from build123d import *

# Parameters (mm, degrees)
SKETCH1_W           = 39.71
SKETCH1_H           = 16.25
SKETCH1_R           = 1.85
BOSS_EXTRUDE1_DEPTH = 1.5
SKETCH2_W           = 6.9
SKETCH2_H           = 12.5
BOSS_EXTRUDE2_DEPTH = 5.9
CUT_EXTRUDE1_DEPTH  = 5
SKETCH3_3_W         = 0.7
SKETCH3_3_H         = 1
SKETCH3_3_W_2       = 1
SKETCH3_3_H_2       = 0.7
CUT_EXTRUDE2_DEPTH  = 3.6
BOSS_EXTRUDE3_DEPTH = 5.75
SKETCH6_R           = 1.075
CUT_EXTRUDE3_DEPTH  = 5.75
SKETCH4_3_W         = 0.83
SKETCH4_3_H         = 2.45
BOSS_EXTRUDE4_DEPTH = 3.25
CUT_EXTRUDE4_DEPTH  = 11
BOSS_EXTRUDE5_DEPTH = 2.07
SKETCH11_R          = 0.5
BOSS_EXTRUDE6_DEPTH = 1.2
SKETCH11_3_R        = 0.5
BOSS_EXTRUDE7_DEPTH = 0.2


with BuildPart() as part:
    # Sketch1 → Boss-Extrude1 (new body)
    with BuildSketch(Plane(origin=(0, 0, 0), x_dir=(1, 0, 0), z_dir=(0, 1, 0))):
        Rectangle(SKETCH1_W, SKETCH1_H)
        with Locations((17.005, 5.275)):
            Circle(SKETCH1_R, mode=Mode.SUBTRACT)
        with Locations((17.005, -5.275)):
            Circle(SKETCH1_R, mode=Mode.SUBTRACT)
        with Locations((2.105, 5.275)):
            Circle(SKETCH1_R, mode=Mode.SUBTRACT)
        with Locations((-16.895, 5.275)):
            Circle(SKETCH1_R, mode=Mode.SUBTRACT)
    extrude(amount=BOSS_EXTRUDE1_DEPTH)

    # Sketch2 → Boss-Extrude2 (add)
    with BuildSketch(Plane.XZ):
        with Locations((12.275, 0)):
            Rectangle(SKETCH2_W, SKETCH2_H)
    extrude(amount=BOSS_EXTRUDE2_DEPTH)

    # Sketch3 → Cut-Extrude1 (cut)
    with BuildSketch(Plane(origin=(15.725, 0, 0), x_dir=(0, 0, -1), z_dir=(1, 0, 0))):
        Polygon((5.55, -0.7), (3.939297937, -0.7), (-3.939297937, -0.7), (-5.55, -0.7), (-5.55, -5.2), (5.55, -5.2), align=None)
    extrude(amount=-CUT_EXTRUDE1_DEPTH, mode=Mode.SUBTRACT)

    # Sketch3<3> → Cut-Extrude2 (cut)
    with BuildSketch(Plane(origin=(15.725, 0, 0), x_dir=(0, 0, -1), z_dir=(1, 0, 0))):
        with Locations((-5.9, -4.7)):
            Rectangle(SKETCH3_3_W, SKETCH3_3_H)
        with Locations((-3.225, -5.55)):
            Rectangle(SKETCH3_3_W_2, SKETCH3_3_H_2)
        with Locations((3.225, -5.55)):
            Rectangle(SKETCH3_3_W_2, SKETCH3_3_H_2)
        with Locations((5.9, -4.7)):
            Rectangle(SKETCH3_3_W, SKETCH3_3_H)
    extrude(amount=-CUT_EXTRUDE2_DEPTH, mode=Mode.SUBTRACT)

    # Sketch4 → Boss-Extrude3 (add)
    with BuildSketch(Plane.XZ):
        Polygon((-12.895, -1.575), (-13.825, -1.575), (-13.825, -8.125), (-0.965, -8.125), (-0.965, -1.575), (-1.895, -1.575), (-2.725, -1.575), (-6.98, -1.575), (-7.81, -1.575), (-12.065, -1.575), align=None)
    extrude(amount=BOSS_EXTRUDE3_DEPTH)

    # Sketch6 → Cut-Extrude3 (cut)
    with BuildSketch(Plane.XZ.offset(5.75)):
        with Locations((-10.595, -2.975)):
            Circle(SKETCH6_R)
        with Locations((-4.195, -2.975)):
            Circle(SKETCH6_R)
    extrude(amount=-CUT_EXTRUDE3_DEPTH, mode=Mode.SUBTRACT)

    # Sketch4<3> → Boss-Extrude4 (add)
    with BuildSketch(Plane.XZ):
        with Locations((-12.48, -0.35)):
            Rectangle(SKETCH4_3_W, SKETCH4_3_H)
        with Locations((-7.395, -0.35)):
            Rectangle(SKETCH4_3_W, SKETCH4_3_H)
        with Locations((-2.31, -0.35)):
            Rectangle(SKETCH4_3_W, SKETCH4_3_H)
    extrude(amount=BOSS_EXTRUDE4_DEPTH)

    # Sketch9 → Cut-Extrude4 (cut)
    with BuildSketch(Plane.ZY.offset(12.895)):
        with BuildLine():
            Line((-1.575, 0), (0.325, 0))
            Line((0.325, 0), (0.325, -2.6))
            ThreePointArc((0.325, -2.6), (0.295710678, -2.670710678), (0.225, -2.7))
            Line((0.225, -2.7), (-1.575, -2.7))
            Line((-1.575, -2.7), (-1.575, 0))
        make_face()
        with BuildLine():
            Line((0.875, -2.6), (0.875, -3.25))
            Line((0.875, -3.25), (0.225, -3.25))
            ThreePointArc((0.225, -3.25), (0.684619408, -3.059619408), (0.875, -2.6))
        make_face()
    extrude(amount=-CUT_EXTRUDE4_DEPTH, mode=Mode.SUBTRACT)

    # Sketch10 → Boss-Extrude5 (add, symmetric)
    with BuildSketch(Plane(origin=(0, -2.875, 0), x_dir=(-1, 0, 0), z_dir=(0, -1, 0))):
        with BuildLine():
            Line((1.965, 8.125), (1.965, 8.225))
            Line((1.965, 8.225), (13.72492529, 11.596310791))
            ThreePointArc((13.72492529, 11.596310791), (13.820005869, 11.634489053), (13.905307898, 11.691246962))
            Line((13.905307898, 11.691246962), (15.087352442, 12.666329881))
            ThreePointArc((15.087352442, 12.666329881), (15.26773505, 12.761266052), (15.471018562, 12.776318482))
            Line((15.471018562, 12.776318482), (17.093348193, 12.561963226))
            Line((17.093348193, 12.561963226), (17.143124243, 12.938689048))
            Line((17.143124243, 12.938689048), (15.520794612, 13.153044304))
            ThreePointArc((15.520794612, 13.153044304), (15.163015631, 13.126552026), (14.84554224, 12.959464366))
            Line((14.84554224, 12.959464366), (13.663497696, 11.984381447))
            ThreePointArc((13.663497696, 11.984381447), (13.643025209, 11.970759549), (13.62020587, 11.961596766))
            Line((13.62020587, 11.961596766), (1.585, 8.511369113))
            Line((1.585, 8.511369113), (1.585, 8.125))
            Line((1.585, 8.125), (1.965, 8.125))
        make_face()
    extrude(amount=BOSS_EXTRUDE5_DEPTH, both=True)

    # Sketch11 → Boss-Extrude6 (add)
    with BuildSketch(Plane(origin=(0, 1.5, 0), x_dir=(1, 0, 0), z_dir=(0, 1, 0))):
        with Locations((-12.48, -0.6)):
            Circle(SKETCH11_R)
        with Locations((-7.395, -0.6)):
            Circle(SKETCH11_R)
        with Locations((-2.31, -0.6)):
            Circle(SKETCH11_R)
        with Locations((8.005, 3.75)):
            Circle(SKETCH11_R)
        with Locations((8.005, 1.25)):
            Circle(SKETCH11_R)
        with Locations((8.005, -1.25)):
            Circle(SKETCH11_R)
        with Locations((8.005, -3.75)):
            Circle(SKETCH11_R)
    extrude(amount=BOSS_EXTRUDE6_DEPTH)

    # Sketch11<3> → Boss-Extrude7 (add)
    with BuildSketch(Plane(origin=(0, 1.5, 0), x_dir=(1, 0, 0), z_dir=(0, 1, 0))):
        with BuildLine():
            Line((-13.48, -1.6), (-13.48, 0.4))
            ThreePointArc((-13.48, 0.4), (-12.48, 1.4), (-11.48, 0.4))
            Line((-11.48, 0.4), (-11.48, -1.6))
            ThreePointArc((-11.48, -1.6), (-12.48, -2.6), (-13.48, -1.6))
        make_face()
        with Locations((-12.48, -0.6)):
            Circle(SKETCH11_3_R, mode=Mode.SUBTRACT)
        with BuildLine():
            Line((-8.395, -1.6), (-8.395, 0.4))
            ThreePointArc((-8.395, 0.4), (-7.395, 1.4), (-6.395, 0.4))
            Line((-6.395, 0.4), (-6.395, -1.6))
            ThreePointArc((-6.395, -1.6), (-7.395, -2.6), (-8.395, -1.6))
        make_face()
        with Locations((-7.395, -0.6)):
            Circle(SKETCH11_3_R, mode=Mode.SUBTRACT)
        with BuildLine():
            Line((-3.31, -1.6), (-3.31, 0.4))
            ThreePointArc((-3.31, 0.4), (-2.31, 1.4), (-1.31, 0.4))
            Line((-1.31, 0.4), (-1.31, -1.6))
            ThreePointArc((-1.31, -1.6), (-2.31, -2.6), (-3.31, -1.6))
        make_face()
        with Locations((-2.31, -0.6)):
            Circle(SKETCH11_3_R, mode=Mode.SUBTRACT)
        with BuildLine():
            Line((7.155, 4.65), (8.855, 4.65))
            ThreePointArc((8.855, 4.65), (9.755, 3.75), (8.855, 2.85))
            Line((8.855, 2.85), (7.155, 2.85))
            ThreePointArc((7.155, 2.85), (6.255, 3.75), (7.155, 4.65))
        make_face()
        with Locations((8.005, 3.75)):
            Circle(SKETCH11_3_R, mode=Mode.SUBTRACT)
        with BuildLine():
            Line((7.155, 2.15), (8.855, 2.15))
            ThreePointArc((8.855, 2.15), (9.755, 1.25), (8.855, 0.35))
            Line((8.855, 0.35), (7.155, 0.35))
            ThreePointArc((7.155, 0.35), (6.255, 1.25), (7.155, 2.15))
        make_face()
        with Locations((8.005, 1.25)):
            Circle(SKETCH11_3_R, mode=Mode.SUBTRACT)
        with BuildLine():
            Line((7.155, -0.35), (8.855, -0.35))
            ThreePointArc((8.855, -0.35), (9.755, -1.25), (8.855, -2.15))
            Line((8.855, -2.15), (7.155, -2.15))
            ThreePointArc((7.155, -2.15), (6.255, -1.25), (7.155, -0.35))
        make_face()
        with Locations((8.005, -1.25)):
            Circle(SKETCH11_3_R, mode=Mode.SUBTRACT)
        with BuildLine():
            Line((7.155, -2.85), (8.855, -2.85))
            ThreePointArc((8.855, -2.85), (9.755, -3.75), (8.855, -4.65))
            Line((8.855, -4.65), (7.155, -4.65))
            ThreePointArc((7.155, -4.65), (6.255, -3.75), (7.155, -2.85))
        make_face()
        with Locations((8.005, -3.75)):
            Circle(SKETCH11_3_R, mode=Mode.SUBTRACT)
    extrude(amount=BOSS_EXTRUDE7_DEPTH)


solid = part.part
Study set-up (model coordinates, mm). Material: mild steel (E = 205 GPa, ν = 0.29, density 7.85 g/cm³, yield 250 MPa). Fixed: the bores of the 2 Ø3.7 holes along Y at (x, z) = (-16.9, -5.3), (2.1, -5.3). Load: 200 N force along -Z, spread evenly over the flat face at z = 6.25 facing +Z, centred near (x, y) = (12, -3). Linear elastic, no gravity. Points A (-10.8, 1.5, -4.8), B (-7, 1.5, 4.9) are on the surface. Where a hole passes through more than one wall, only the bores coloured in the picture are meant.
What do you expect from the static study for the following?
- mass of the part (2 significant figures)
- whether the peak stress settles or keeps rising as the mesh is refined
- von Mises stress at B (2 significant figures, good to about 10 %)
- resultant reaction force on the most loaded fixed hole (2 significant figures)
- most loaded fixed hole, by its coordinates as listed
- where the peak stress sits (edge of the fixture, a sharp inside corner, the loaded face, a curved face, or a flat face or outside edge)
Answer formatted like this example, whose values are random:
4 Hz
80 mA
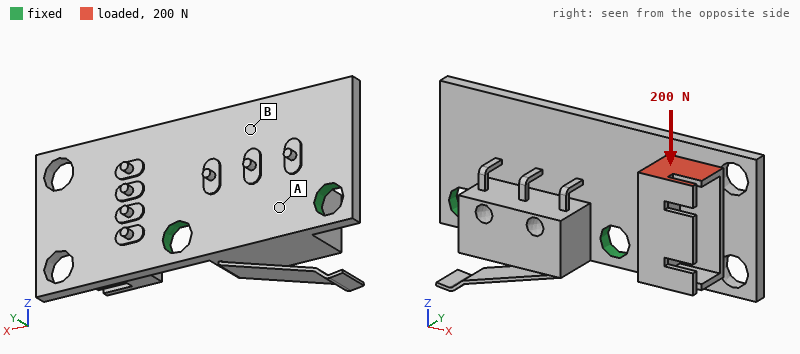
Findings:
13 g
keeps rising
31 MPa
280 N
(2.1, -5.3)
edge of the fixture
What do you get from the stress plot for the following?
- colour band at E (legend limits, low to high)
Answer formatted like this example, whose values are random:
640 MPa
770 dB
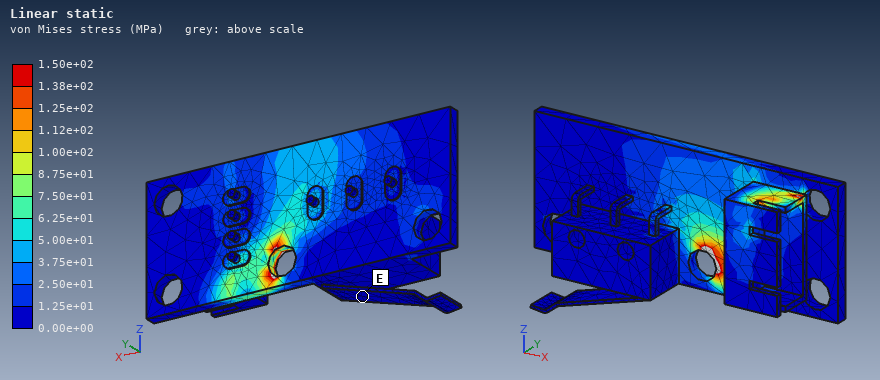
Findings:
0.00e+00 to 1.25e+01 MPa
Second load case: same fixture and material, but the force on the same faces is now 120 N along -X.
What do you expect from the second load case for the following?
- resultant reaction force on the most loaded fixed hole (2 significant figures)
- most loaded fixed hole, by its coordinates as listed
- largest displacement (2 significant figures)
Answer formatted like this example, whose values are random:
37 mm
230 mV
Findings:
88 N
(-16.9, -5.3)
55 µm
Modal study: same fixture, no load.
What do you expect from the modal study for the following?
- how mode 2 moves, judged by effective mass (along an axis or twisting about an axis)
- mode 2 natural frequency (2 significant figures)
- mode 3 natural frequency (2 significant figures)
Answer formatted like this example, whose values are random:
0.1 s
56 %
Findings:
along Y
3300 Hz
7000 Hz
